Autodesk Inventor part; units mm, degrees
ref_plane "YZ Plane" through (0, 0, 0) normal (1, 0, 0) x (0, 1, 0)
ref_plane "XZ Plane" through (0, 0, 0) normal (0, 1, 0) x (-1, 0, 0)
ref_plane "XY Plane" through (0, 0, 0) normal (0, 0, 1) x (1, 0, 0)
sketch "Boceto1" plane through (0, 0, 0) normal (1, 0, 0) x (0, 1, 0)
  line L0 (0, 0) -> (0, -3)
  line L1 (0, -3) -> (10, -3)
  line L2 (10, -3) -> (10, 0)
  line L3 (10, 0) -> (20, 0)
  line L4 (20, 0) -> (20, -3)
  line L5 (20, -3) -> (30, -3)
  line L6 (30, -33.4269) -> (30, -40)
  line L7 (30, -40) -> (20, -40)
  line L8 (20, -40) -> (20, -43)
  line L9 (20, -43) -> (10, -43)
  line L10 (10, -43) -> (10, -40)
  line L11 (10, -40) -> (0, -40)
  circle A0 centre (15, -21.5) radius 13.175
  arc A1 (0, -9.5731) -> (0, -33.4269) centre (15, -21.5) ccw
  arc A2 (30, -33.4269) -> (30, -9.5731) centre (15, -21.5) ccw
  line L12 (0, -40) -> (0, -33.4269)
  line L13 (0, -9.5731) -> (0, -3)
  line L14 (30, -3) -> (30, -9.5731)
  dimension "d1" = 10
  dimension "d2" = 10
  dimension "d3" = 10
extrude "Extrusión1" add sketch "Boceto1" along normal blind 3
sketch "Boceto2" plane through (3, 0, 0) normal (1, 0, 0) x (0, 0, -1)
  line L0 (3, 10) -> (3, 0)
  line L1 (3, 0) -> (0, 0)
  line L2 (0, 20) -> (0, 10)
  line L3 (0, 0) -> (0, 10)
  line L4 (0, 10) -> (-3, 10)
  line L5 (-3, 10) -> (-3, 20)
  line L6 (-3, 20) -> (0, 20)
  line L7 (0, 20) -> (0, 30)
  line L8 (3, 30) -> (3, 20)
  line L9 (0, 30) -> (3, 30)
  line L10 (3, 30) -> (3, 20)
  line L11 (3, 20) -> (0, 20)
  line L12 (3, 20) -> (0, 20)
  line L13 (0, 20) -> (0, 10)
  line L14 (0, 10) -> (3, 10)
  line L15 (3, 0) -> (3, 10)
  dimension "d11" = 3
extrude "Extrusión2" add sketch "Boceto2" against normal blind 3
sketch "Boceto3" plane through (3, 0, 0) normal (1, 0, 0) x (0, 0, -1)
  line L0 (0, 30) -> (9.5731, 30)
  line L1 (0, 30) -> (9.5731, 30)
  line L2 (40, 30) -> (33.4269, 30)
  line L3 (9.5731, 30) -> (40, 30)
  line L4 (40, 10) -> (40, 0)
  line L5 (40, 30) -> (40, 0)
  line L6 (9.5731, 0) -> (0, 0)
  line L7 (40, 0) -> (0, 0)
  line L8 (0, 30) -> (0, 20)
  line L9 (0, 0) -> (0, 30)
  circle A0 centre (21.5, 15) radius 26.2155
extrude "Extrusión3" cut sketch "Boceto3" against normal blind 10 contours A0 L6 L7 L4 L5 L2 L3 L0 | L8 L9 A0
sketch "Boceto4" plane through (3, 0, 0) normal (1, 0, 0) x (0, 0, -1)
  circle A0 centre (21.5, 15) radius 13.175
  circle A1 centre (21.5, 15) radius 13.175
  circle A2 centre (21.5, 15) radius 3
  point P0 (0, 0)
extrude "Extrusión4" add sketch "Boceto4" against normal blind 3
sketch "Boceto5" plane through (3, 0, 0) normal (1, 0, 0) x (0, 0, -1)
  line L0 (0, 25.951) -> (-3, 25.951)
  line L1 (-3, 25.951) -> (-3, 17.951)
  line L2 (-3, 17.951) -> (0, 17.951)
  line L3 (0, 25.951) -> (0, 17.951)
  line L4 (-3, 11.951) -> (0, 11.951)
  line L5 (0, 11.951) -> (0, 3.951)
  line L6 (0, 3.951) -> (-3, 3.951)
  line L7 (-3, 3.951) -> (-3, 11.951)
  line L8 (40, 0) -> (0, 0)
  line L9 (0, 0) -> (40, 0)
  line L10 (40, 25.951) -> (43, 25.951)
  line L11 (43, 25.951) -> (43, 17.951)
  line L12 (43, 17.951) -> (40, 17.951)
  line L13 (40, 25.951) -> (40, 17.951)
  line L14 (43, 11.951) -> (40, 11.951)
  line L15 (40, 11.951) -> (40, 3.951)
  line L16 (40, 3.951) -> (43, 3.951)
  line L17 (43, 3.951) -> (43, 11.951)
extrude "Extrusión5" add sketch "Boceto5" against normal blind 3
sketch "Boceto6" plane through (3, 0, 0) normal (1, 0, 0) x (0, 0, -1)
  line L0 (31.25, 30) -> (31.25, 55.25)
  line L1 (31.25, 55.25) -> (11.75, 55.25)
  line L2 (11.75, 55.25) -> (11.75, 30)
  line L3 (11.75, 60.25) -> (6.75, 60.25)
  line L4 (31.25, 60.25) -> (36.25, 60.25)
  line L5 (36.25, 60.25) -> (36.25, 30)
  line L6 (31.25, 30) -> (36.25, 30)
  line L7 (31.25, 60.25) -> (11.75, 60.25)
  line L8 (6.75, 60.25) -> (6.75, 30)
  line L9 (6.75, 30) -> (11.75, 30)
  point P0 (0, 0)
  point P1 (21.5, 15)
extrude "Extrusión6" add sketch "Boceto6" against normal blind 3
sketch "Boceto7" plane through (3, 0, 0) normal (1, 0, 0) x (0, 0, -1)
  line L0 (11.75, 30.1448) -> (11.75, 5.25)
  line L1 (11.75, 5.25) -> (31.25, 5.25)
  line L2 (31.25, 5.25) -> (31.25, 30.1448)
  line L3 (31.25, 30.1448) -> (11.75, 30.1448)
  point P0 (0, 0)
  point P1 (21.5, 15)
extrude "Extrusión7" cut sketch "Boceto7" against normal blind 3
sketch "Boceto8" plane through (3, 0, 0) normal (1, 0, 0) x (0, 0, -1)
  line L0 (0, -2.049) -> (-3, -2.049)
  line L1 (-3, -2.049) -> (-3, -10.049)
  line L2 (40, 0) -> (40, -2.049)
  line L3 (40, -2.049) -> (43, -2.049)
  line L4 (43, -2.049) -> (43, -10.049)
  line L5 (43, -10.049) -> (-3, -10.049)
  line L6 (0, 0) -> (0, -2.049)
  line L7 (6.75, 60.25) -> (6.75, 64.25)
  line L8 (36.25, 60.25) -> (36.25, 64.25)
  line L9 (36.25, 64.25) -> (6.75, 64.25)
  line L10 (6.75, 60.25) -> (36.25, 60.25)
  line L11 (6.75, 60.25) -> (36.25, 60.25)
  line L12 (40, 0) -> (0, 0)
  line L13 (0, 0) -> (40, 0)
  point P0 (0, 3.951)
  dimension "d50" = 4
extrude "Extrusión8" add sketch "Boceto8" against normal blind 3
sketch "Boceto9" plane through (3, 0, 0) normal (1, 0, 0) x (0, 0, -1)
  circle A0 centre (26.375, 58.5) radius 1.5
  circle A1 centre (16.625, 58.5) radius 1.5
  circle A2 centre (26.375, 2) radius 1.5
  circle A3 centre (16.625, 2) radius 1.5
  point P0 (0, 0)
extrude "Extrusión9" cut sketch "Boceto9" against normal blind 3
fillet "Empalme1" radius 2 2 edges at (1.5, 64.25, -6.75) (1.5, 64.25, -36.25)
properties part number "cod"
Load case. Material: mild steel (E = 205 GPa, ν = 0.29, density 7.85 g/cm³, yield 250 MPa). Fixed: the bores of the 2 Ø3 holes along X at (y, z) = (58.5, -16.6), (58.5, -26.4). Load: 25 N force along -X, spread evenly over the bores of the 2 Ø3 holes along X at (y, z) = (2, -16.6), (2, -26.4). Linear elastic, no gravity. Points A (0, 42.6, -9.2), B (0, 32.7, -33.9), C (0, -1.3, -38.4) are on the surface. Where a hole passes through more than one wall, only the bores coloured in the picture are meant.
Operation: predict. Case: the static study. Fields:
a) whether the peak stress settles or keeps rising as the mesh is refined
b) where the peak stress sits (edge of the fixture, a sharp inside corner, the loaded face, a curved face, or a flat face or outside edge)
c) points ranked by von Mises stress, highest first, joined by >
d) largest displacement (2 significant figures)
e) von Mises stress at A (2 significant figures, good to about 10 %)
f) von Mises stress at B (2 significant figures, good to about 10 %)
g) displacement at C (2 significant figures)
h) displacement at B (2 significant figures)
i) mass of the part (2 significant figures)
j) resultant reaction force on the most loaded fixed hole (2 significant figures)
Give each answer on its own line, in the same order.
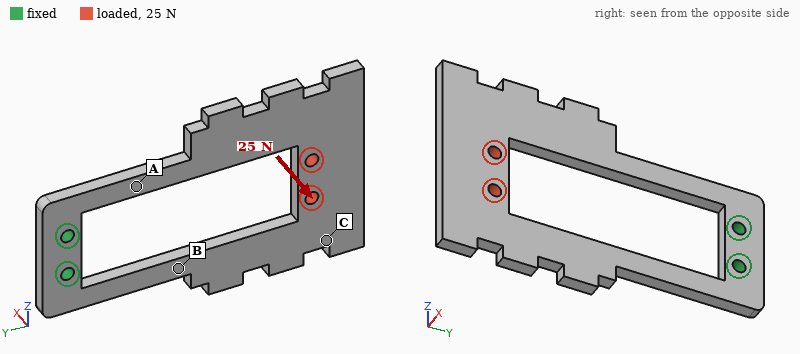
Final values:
keeps rising
a sharp inside corner
A > B > C
0.44 mm
68 MPa
51 MPa
0.37 mm
0.100 mm
41 g
13 N
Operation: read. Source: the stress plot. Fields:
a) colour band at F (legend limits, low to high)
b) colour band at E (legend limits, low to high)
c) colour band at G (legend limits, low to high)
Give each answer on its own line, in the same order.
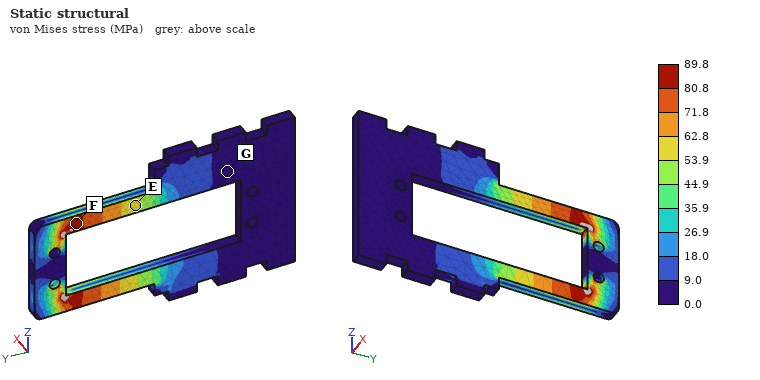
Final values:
80.8 to 89.8 MPa
53.9 to 62.8 MPa
0.0 to 9.0 MPa
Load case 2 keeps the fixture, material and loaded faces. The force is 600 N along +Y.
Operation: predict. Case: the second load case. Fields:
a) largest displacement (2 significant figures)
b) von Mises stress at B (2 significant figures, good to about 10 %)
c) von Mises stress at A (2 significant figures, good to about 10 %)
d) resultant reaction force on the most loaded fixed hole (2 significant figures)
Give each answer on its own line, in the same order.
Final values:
9.2 µm
20 MPa
20 MPa
330 N
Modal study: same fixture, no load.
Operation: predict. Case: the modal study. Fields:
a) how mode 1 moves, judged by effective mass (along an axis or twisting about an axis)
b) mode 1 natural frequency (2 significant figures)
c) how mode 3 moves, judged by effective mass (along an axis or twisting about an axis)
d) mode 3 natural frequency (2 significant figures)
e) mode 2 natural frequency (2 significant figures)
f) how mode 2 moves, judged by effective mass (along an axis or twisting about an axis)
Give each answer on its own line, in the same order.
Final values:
along X
270 Hz
along Z
1100 Hz
850 Hz
twisting about Y
